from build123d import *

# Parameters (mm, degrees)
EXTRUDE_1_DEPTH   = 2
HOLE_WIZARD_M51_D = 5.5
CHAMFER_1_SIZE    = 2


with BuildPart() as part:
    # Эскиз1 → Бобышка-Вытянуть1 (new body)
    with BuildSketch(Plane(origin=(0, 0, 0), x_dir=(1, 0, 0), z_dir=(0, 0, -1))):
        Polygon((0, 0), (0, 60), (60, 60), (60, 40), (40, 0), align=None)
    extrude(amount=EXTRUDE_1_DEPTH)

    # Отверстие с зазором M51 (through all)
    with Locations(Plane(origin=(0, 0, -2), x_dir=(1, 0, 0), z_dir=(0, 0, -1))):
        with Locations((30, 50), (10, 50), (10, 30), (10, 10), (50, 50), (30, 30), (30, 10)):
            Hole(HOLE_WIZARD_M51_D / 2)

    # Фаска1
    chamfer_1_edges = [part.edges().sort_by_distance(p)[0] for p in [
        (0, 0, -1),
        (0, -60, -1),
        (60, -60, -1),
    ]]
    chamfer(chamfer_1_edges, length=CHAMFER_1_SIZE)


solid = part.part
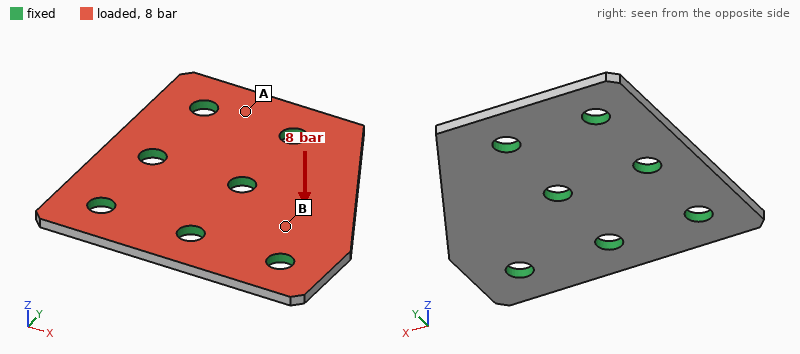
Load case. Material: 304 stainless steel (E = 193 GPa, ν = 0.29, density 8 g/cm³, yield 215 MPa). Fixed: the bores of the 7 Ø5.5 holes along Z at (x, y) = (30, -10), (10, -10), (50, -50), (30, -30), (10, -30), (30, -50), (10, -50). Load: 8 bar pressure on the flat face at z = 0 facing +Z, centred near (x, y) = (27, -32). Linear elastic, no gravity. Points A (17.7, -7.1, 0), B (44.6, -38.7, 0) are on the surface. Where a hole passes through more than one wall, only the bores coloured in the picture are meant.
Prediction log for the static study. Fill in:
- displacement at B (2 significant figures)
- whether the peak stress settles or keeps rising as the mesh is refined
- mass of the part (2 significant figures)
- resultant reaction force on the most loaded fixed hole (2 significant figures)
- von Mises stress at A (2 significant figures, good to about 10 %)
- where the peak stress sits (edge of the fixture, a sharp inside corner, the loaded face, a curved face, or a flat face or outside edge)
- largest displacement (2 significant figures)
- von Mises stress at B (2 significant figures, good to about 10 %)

14 µm
keeps rising
48 g
430 N
16 MPa
edge of the fixture
62 µm
56 MPa
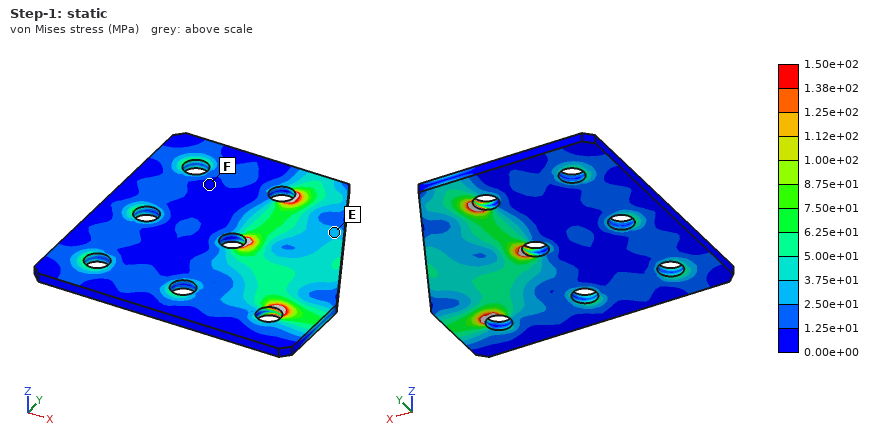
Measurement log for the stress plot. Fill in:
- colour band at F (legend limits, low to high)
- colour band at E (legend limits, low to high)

0.00e+00 to 1.25e+01 MPa
2.50e+01 to 3.75e+01 MPa
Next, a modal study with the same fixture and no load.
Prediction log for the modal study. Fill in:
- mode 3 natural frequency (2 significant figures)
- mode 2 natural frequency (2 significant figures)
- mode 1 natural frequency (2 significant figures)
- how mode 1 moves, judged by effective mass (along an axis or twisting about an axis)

16 kHz
12 kHz
6200 Hz
along Z
